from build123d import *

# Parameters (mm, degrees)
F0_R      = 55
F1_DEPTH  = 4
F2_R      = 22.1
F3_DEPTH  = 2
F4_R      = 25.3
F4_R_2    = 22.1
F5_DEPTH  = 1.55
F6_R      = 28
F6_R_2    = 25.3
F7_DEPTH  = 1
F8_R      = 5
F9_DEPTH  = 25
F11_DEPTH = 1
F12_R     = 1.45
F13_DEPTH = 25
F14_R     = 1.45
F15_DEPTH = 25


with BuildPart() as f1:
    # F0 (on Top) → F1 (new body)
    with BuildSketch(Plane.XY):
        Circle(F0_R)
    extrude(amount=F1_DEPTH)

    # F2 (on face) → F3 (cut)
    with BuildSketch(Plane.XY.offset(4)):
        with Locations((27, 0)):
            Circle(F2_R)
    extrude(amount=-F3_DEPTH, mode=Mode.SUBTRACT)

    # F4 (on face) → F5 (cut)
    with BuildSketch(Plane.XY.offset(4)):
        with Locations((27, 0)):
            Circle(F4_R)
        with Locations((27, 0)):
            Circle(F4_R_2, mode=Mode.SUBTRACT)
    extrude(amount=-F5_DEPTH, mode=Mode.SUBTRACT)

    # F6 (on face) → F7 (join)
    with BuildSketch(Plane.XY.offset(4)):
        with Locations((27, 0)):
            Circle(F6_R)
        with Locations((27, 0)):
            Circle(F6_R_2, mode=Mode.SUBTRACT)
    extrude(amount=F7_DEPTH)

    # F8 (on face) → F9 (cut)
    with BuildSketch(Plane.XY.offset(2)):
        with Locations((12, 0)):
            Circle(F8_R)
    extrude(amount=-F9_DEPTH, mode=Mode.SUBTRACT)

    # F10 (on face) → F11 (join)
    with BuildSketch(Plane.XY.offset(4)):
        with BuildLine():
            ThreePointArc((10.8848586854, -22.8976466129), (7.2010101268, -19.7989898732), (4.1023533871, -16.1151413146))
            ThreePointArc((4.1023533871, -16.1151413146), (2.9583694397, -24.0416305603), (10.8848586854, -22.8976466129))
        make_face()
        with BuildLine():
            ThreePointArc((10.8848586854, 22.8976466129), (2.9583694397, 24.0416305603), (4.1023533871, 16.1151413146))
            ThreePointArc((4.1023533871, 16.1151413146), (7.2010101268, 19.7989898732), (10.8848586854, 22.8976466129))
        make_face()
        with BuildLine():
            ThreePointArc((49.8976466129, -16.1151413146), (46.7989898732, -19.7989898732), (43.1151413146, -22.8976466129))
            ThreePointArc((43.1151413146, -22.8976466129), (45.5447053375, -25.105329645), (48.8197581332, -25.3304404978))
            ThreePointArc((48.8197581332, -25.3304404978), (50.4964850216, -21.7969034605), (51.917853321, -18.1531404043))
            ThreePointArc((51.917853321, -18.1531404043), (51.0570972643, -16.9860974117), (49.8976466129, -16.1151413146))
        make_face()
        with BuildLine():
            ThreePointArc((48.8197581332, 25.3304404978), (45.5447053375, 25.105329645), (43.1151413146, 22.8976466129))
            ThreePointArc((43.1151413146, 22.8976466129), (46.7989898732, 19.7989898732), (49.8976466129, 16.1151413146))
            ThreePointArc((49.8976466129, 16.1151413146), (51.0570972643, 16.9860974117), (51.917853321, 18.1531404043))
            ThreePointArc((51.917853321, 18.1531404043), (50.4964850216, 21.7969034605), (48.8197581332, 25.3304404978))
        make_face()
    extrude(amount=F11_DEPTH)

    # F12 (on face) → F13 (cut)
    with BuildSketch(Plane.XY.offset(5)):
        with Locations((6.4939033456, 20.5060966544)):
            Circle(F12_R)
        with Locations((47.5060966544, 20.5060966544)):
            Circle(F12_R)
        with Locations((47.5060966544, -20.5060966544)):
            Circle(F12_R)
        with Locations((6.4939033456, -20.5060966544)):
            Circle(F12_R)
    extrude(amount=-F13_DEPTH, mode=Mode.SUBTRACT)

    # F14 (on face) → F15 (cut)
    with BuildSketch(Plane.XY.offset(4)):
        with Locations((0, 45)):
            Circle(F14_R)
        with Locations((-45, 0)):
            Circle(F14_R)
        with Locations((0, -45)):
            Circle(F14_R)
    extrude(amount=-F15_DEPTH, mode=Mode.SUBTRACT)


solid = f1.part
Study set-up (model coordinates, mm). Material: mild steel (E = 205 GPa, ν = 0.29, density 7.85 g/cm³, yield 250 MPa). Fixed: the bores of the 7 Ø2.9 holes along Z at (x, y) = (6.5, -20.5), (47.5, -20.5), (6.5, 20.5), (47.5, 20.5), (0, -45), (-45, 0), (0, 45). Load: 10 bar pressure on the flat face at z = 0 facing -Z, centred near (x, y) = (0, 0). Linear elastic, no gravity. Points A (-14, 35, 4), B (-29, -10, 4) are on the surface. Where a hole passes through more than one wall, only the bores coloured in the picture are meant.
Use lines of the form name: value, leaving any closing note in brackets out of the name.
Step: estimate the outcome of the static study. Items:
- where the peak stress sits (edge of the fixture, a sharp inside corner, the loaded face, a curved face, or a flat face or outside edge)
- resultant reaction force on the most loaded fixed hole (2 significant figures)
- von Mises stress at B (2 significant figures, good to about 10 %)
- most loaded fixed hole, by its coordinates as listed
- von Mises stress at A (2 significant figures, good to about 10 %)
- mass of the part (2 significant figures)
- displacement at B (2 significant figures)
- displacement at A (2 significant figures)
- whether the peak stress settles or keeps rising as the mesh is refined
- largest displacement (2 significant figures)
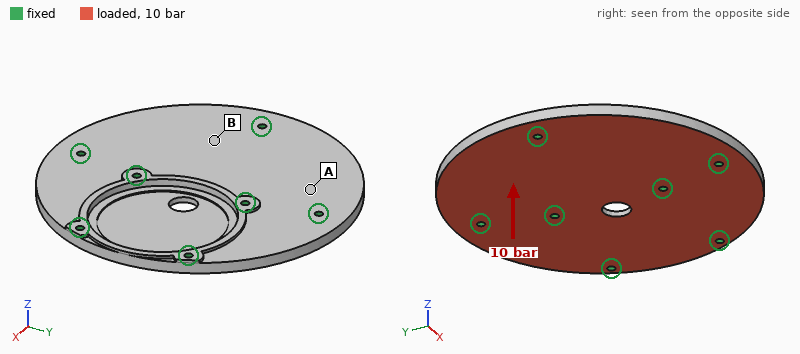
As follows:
where the peak stress sits: edge of the fixture
resultant reaction force on the most loaded fixed hole: 2.0 kN
von Mises stress at B: 66 MPa
most loaded fixed hole, by its coordinates as listed: (-45, 0)
von Mises stress at A: 33 MPa
mass of the part: 270 g
displacement at B: 29 µm
displacement at A: 29 µm
whether the peak stress settles or keeps rising as the mesh is refined: keeps rising
largest displacement: 86 µm
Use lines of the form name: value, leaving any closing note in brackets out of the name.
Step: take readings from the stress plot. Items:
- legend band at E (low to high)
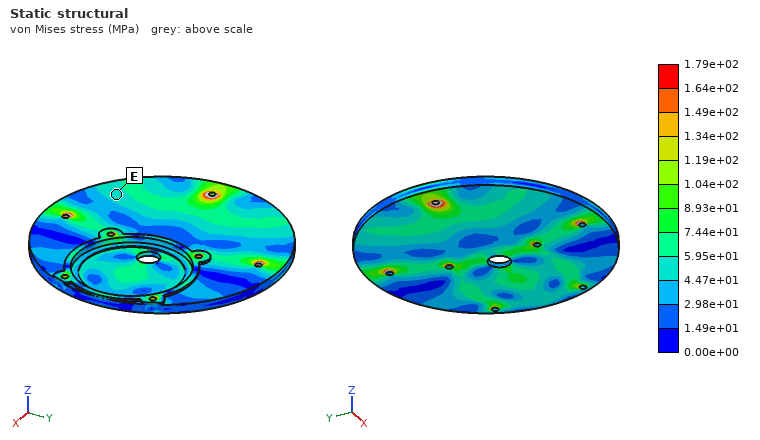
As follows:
legend band at E: 4.47e+01 to 5.95e+01 MPa
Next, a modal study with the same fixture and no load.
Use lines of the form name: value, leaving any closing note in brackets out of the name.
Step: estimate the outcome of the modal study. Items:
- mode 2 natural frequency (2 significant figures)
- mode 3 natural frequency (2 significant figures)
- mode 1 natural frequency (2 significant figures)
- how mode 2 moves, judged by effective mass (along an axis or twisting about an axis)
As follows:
mode 2 natural frequency: 4000 Hz
mode 3 natural frequency: 6700 Hz
mode 1 natural frequency: 3600 Hz
how mode 2 moves, judged by effective mass: along Z
